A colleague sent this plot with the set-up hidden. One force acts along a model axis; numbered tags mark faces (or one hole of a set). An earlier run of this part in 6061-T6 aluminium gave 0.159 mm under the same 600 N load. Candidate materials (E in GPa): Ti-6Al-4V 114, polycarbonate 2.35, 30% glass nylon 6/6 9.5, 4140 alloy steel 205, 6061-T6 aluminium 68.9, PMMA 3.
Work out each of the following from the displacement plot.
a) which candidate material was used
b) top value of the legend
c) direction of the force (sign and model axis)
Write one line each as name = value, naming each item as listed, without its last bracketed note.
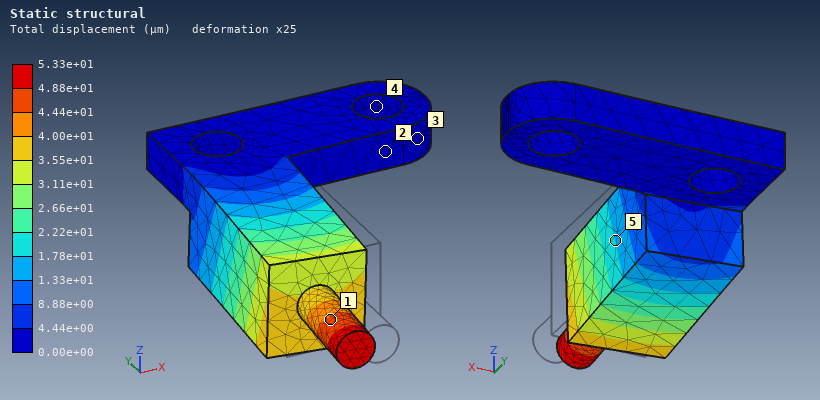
which candidate material was used = 4140 alloy steel
top value of the legend = 5.33e+01 µm
direction of the force = -X
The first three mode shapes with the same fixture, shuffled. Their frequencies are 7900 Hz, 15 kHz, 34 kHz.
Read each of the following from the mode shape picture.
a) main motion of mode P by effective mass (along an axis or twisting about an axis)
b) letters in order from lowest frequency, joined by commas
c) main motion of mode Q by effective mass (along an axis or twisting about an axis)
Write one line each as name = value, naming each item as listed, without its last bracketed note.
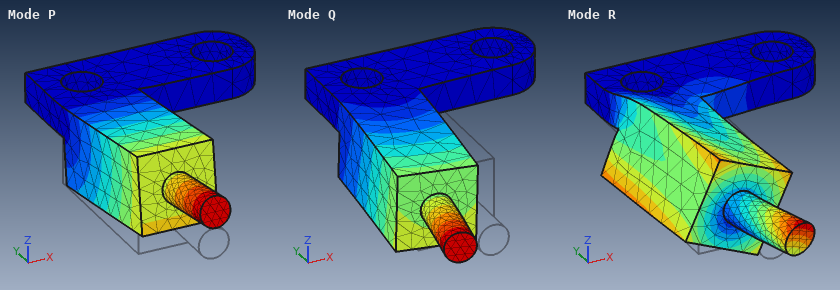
main motion of mode P by effective mass = along Z
letters in order from lowest frequency, joined by commas = P, Q, R
main motion of mode Q by effective mass = along X
